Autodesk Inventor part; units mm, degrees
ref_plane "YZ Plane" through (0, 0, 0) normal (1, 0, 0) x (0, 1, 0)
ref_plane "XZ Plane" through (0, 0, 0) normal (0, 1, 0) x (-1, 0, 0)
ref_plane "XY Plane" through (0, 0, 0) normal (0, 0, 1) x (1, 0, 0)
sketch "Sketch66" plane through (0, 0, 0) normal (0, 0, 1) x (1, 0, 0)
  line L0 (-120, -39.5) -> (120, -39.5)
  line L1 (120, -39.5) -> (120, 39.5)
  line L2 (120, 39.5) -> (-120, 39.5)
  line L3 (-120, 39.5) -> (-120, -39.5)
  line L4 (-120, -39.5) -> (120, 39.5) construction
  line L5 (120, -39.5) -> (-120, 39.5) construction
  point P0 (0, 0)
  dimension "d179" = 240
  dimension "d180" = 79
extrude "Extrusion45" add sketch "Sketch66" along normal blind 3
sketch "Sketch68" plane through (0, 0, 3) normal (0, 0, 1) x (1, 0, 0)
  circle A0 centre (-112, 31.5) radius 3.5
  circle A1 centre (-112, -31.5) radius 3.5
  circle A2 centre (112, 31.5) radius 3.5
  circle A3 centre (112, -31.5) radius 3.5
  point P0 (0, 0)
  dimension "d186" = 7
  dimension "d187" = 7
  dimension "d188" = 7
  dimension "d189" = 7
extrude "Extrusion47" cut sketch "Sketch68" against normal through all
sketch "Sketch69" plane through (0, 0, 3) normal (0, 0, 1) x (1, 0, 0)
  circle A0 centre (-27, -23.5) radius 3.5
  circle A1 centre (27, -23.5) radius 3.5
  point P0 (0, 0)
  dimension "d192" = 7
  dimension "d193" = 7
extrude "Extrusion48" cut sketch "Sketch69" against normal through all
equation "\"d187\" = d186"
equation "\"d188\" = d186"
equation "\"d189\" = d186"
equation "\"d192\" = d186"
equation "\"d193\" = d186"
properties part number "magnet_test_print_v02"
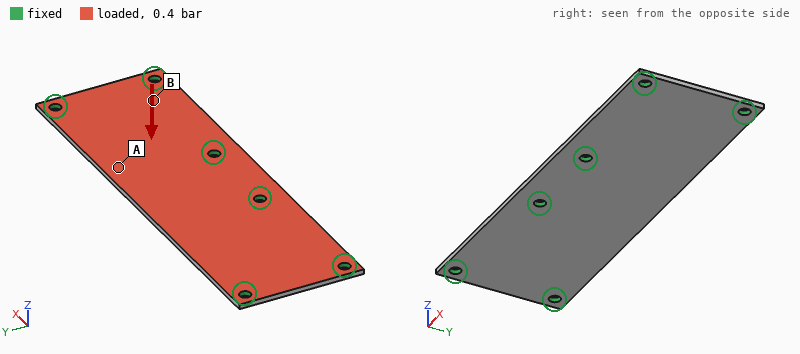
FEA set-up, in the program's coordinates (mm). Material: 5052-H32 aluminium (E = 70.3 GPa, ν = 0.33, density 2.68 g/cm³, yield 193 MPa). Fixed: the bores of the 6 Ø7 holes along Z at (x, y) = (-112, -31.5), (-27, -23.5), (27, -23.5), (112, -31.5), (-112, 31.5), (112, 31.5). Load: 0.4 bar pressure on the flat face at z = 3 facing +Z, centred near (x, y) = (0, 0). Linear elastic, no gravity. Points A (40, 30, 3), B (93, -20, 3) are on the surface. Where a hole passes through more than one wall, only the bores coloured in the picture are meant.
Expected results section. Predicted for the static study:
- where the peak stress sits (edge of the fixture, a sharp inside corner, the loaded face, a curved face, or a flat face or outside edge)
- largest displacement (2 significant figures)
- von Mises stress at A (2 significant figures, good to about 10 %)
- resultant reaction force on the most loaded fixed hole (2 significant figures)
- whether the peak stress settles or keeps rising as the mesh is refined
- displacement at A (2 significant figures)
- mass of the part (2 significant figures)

edge of the fixture
0.36 mm
13 MPa
200 N
keeps rising
0.25 mm
150 g
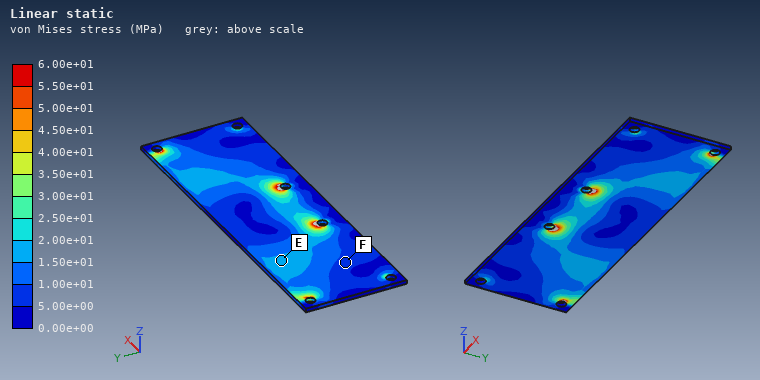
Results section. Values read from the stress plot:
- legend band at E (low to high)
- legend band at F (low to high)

1.50e+01 to 2.00e+01 MPa
5.00e+00 to 1.00e+01 MPa
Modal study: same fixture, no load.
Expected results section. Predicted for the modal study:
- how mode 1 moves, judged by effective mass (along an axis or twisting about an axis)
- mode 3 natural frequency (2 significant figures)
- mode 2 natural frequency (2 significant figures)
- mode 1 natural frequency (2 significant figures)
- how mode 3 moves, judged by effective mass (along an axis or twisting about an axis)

along Z
1900 Hz
1300 Hz
800 Hz
along Z
